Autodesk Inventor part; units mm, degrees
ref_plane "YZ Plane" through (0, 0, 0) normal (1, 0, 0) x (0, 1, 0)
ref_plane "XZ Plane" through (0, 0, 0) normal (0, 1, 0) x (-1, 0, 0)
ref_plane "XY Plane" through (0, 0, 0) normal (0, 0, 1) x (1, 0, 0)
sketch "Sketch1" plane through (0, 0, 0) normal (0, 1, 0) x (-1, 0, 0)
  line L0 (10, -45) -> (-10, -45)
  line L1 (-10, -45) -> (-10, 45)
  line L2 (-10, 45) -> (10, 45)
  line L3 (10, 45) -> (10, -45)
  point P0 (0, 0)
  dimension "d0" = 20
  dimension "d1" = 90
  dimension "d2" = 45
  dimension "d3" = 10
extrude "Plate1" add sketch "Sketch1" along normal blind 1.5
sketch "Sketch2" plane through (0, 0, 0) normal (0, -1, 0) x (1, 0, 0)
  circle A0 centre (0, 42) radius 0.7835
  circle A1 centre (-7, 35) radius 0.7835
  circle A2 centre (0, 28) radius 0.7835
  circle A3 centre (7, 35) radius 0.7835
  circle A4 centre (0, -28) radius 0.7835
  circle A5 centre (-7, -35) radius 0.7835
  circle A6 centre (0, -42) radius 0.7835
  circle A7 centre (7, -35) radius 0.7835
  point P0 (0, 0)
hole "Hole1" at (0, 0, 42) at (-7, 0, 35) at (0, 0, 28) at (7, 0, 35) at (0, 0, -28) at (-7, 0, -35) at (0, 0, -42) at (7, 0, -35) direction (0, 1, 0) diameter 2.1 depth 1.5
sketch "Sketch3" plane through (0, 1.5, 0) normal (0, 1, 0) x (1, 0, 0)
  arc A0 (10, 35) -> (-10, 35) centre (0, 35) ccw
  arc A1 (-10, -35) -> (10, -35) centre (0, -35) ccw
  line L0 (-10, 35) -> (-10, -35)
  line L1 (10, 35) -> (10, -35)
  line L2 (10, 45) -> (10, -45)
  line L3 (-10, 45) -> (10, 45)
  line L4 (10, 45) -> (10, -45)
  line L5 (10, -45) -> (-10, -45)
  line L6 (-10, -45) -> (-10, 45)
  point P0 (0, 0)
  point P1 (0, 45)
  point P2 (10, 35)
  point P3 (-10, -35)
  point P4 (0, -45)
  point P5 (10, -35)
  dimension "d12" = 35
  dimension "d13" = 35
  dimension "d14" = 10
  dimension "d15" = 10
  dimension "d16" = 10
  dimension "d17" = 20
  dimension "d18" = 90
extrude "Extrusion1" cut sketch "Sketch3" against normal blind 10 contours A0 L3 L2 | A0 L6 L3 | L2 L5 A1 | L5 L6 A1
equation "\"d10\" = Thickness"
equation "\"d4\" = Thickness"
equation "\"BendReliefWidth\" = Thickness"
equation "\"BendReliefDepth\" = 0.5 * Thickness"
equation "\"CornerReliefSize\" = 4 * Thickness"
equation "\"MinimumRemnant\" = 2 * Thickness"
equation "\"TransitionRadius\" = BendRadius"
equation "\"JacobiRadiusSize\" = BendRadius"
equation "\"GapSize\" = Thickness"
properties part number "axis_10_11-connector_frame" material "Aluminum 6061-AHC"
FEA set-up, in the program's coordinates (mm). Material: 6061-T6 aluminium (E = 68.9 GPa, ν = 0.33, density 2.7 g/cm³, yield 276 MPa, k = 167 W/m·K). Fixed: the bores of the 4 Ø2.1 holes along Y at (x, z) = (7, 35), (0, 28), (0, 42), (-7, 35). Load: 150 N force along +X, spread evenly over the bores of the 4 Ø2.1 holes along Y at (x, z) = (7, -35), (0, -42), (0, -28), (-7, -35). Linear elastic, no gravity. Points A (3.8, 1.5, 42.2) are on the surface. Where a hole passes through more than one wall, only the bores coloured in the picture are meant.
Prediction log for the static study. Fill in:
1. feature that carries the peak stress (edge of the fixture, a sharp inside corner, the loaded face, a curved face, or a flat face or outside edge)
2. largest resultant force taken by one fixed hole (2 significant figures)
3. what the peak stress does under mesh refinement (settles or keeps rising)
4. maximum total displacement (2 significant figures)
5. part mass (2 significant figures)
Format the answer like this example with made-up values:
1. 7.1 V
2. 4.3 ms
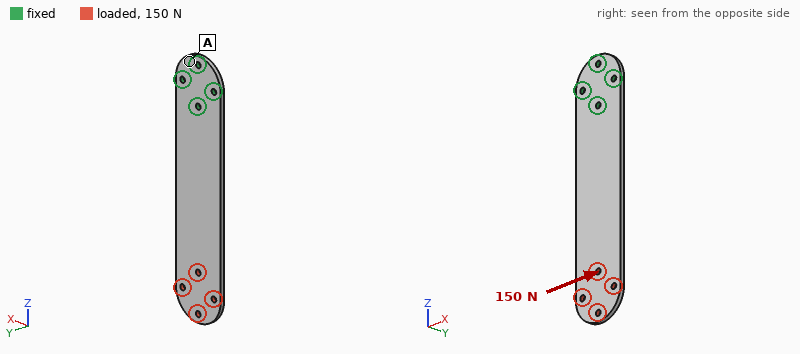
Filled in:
1. edge of the fixture
2. 500 N
3. keeps rising
4. 0.31 mm
5. 6.8 g
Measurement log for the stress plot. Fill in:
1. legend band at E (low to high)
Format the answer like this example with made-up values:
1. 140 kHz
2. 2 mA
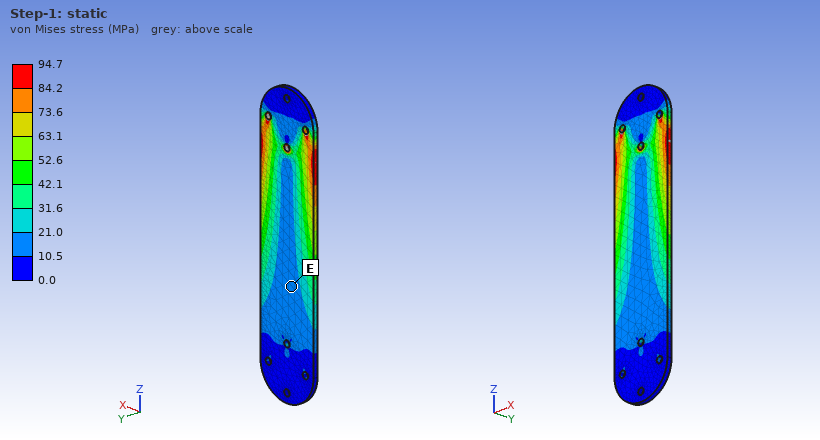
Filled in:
1. 10.5 to 21.0 MPa
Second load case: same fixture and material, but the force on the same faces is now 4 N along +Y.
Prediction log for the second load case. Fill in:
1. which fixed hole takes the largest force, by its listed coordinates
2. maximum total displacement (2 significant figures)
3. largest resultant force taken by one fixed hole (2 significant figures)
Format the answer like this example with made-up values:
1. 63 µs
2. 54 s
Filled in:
1. (0, 28)
2. 1.1 mm
3. 24 N
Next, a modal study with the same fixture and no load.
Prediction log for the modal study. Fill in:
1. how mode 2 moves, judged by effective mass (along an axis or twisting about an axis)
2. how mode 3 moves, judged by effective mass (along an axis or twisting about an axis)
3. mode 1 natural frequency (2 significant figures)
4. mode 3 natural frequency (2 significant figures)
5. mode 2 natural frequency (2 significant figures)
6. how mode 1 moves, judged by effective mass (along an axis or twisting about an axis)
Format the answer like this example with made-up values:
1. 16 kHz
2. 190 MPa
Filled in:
1. along Y
2. twisting about Z
3. 250 Hz
4. 1700 Hz
5. 1500 Hz
6. along Y
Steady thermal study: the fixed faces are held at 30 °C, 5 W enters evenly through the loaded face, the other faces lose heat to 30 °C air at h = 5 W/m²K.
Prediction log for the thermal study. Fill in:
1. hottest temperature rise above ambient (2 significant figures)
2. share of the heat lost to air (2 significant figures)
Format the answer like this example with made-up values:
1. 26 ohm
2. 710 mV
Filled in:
1. 62 K
2. 10 %
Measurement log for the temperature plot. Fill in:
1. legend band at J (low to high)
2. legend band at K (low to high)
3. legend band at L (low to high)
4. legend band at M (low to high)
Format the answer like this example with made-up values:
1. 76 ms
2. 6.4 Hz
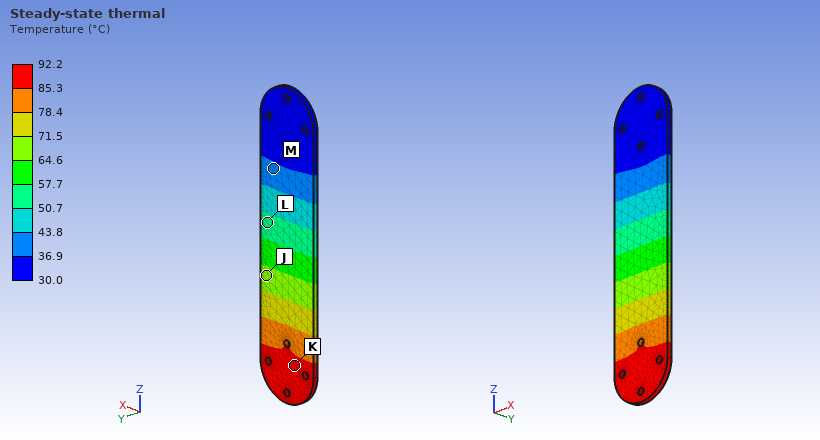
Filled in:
1. 64.6 to 71.5 °C
2. 85.3 to 92.2 °C
3. 50.7 to 57.7 °C
4. 36.9 to 43.8 °C
